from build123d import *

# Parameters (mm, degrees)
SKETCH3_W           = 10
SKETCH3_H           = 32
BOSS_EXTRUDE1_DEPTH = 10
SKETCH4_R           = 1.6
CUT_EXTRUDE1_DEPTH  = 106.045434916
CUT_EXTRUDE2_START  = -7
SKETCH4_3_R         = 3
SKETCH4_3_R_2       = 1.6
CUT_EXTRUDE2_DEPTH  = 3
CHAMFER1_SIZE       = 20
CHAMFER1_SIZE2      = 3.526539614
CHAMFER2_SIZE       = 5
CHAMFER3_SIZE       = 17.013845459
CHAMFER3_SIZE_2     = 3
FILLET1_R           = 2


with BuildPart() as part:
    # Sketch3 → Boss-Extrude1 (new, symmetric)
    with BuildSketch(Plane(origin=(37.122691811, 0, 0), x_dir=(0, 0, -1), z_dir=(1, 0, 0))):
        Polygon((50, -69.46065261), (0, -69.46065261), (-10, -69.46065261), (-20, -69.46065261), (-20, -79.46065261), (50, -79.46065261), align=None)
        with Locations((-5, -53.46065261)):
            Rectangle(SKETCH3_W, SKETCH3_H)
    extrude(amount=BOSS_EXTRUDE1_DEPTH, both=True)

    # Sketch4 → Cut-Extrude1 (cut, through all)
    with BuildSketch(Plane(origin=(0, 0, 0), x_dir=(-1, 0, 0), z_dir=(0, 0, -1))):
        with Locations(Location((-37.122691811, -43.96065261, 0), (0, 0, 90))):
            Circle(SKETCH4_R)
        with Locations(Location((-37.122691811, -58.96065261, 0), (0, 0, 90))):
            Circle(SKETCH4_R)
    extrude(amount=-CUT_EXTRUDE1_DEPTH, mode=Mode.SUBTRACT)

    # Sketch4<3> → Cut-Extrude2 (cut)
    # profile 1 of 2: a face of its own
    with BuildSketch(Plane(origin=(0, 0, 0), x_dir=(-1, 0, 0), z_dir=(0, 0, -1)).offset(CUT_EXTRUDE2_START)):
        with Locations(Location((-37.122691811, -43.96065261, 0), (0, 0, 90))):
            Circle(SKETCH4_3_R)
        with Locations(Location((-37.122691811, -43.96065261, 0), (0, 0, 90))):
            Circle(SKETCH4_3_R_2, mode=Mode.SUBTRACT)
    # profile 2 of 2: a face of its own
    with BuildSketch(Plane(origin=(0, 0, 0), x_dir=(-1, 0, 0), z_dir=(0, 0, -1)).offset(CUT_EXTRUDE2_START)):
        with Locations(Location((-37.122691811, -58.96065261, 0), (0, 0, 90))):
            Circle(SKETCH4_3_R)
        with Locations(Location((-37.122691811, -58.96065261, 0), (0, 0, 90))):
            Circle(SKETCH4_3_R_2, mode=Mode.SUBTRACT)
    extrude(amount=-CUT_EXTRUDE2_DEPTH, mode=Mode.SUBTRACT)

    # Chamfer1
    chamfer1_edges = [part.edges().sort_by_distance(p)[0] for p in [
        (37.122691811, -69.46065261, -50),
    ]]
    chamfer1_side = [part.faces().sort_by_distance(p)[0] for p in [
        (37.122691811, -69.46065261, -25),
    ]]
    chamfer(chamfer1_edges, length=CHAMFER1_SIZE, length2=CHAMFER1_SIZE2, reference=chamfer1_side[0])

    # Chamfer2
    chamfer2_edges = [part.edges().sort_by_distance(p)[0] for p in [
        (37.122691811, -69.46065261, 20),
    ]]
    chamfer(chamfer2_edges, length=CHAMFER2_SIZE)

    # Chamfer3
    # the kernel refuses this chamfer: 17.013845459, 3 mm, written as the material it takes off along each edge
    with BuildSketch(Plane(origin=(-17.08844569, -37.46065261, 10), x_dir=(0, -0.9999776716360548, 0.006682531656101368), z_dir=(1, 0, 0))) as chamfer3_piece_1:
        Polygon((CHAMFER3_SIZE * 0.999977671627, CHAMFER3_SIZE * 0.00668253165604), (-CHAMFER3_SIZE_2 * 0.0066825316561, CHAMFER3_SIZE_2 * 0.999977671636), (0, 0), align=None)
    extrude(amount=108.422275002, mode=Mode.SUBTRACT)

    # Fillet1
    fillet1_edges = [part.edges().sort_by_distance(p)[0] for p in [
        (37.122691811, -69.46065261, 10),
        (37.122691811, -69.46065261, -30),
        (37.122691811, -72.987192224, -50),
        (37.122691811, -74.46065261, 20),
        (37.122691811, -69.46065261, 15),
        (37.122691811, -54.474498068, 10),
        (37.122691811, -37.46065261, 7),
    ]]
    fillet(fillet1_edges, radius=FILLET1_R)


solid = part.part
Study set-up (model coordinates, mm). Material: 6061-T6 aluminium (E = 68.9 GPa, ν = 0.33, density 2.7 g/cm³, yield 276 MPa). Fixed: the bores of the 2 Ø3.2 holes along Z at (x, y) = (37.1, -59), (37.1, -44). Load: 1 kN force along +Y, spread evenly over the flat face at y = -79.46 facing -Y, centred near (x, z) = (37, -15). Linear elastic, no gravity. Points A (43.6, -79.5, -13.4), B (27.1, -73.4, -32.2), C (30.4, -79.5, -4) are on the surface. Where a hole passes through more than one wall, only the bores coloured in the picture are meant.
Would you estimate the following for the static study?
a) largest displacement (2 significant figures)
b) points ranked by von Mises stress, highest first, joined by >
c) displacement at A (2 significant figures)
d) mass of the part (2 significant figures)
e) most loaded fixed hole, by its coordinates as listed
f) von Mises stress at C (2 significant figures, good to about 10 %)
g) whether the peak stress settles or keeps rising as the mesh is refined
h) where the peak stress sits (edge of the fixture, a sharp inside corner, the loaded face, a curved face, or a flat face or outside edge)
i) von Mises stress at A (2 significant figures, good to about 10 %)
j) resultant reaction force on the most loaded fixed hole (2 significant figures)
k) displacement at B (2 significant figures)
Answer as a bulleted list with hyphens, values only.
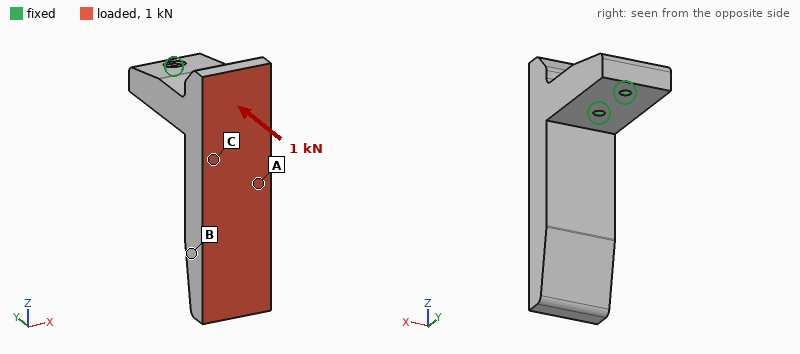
- 0.30 mm
- C > A > B
- 0.096 mm
- 50 g
- (37.1, -59)
- 45 MPa
- keeps rising
- edge of the fixture
- 29 MPa
- 1.4 kN
- 0.19 mm
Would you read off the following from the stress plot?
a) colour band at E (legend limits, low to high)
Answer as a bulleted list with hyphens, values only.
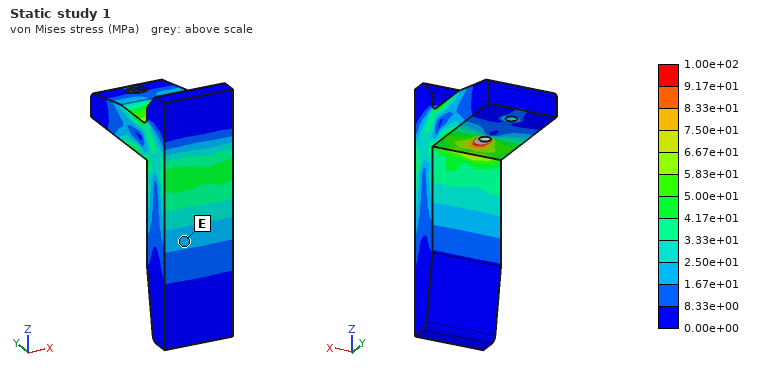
- 1.67e+01 to 2.50e+01 MPa
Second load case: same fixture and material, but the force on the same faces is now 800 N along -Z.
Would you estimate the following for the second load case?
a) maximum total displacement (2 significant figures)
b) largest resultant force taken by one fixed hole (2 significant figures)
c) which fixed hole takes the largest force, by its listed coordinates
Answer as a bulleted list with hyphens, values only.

- 0.14 mm
- 1.4 kN
- (37.1, -59)
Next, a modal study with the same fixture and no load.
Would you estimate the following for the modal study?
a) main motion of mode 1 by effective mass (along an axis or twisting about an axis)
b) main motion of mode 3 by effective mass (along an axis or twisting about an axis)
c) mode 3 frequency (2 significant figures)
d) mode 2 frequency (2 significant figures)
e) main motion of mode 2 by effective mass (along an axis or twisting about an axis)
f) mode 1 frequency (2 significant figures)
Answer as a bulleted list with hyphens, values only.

- along Y
- along Z
- 7000 Hz
- 2300 Hz
- along X
- 1900 Hz
